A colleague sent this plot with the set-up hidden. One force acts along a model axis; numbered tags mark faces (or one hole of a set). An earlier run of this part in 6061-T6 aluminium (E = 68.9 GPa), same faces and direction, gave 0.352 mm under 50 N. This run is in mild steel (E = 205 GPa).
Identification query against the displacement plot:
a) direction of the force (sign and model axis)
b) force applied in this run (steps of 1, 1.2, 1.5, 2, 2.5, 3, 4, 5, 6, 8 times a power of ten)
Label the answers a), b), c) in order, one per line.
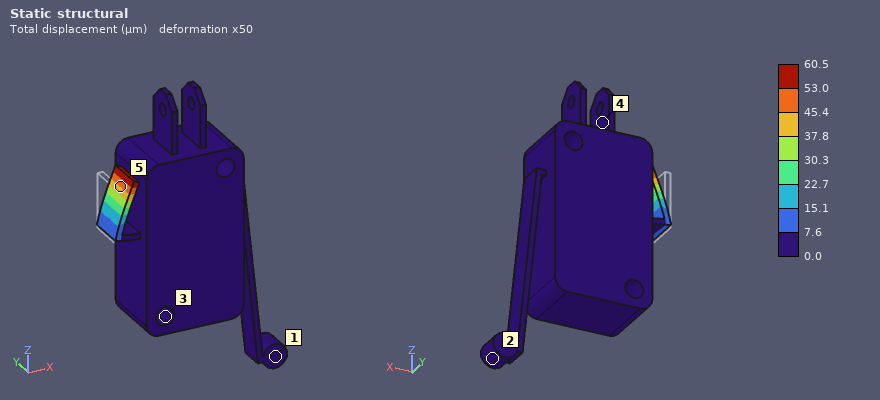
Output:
a) +X
b) 25 N
